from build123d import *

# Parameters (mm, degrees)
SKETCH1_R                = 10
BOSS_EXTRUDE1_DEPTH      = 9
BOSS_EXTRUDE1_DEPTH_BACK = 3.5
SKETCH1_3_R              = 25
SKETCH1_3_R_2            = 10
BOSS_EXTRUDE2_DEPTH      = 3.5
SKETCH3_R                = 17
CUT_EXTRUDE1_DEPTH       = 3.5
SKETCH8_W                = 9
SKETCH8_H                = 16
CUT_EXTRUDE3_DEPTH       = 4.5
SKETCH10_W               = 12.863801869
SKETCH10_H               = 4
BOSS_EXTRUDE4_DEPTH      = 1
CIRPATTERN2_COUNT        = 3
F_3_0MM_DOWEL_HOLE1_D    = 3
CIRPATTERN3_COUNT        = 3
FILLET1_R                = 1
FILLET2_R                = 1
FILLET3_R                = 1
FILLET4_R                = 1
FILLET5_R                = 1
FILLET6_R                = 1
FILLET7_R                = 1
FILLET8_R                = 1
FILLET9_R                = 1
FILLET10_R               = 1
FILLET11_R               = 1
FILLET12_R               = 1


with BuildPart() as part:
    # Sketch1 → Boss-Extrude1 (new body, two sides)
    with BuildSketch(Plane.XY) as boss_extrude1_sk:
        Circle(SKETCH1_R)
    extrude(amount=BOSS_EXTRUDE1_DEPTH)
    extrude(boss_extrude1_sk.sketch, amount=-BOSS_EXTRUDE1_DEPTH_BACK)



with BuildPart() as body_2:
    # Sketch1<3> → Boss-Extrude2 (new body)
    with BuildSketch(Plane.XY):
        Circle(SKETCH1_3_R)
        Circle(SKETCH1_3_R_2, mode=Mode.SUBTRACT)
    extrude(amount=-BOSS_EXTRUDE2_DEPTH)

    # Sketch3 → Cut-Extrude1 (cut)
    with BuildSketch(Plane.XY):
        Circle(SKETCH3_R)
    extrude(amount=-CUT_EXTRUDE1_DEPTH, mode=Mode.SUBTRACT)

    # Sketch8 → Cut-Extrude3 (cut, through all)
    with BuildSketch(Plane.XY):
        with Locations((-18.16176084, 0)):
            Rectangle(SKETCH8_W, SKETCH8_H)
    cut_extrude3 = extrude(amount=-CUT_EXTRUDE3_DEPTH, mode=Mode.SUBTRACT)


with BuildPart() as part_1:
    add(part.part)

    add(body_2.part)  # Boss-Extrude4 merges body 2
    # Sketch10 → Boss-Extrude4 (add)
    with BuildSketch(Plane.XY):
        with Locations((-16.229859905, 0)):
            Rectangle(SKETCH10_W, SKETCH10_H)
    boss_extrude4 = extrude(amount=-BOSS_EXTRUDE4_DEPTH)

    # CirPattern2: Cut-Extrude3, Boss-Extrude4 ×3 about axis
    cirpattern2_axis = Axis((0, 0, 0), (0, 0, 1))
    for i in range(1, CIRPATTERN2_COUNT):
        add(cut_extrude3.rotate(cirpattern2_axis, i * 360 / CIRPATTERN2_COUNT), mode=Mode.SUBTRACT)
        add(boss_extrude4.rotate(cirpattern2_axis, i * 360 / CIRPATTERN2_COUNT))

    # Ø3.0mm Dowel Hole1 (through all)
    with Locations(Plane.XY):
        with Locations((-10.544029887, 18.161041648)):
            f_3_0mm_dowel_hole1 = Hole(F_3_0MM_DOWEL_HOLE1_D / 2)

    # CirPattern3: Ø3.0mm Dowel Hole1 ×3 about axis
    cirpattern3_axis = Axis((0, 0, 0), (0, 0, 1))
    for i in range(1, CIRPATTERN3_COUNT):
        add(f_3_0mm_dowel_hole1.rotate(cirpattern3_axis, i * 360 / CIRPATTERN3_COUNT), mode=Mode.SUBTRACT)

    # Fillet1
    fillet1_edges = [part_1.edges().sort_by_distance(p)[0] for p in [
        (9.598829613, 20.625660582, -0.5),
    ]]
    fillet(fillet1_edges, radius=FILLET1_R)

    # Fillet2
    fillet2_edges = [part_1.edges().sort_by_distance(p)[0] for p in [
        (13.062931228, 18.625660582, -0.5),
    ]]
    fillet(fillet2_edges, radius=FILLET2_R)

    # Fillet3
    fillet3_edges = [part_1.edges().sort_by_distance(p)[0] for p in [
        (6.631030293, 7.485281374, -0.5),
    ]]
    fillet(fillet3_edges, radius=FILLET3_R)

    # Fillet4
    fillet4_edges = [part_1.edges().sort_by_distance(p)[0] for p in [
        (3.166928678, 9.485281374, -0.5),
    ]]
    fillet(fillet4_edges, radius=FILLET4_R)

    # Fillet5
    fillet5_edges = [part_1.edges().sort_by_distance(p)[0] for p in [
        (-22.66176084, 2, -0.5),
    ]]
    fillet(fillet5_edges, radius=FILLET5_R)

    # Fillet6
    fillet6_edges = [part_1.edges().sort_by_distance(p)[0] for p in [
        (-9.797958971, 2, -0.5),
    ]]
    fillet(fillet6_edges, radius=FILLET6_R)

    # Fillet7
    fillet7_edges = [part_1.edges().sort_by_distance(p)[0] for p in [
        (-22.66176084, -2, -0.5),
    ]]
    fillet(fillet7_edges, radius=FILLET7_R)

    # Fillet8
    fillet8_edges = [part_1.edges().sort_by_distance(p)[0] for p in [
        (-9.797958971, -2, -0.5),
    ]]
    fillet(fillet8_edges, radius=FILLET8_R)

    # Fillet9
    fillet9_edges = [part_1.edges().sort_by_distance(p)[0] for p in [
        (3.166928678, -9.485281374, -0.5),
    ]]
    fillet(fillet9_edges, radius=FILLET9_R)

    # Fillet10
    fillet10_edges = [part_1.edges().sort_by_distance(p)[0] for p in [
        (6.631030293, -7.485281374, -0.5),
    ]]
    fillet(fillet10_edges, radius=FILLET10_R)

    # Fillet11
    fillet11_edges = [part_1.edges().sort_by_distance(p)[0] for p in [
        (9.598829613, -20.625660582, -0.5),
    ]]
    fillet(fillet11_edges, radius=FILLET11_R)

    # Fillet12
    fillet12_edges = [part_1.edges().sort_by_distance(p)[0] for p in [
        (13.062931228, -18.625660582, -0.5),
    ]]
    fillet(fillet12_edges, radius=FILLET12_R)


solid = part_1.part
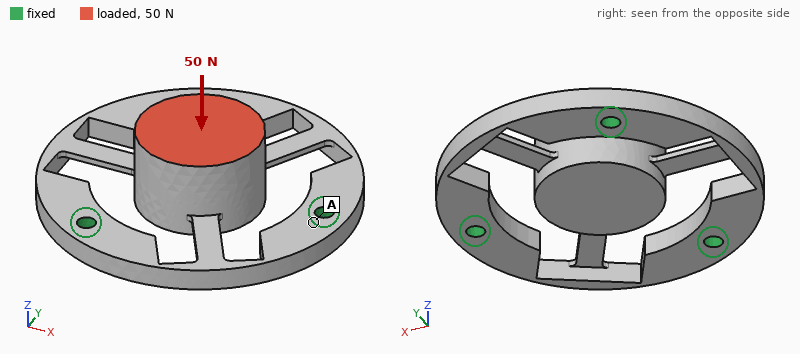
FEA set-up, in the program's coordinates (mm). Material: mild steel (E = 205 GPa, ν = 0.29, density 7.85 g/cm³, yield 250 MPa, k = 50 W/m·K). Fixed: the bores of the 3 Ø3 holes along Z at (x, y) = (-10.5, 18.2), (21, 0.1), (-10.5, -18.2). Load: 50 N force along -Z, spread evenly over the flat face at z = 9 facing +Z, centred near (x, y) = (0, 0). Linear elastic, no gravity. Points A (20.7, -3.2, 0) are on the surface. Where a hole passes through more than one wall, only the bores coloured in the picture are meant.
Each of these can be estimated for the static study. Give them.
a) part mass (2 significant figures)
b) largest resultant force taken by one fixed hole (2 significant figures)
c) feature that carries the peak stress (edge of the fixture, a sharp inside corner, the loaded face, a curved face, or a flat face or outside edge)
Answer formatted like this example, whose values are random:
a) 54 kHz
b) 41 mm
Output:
a) 52 g
b) 18 N
c) a curved face
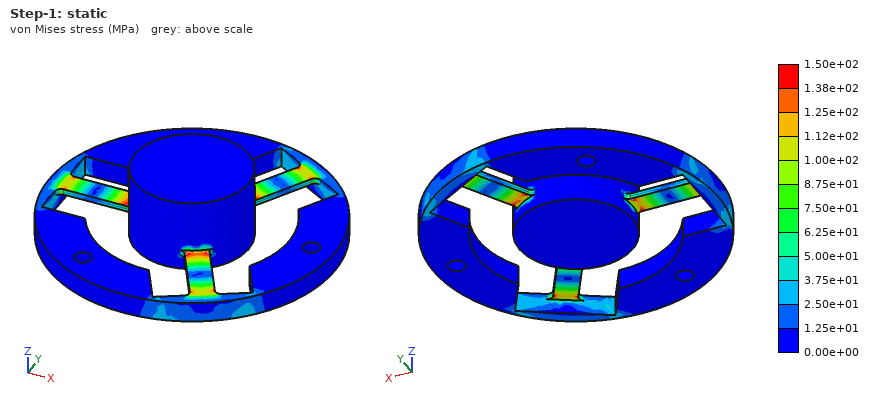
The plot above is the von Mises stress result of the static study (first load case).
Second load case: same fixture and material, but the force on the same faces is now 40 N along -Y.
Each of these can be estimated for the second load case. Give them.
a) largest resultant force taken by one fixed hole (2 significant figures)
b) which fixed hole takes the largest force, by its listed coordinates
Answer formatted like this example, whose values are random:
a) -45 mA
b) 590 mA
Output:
a) 27 N
b) (21, 0.1)
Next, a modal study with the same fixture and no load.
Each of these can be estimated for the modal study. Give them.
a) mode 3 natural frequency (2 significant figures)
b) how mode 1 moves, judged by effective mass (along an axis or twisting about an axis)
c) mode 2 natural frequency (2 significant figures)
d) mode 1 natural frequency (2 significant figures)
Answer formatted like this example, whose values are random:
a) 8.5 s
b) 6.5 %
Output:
a) 1500 Hz
b) along Z
c) 1500 Hz
d) 850 Hz
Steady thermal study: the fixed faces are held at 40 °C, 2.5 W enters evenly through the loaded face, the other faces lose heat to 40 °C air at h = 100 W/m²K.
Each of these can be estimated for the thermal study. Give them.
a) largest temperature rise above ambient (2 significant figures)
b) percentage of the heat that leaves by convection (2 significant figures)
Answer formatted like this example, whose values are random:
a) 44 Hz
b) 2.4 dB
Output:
a) 17 K
b) 88 %
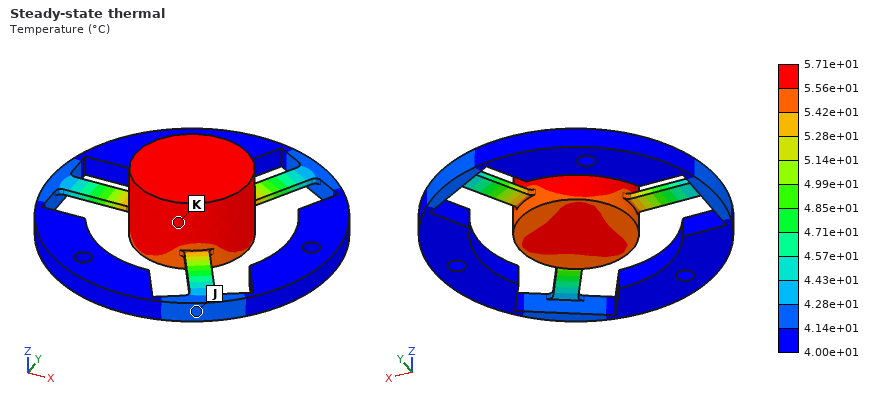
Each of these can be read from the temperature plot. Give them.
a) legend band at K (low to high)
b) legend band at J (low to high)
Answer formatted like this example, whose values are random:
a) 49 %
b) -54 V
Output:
a) 5.56e+01 to 5.71e+01 °C
b) 4.14e+01 to 4.28e+01 °C
